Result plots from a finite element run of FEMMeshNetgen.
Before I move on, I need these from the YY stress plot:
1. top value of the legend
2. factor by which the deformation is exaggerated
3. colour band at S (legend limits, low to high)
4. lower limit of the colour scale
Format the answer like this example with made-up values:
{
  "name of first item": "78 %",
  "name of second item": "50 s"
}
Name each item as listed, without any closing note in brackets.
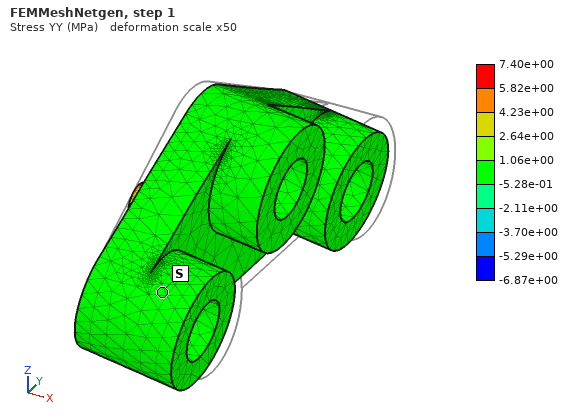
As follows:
{
  "top value of the legend": "7.40e+00 MPa",
  "factor by which the deformation is exaggerated": "50",
  "colour band at S": "-5.28e-01 to 1.06e+00 MPa",
  "lower limit of the colour scale": "-6.87e+00 MPa"
}
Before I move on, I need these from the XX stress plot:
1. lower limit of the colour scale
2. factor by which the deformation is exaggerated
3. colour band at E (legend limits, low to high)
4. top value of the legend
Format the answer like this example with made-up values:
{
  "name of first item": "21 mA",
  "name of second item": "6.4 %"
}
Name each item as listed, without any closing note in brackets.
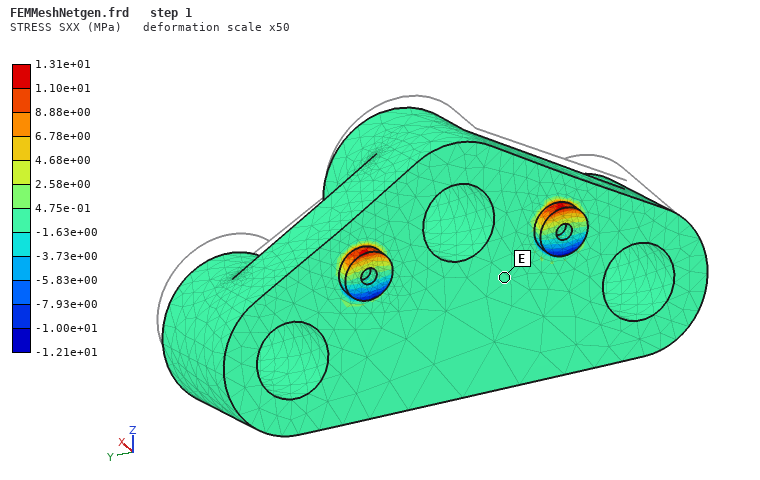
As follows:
{
  "lower limit of the colour scale": "-1.21e+01 MPa",
  "factor by which the deformation is exaggerated": "50",
  "colour band at E": "-1.63e+00 to 4.75e-01 MPa",
  "top value of the legend": "1.31e+01 MPa"
}
